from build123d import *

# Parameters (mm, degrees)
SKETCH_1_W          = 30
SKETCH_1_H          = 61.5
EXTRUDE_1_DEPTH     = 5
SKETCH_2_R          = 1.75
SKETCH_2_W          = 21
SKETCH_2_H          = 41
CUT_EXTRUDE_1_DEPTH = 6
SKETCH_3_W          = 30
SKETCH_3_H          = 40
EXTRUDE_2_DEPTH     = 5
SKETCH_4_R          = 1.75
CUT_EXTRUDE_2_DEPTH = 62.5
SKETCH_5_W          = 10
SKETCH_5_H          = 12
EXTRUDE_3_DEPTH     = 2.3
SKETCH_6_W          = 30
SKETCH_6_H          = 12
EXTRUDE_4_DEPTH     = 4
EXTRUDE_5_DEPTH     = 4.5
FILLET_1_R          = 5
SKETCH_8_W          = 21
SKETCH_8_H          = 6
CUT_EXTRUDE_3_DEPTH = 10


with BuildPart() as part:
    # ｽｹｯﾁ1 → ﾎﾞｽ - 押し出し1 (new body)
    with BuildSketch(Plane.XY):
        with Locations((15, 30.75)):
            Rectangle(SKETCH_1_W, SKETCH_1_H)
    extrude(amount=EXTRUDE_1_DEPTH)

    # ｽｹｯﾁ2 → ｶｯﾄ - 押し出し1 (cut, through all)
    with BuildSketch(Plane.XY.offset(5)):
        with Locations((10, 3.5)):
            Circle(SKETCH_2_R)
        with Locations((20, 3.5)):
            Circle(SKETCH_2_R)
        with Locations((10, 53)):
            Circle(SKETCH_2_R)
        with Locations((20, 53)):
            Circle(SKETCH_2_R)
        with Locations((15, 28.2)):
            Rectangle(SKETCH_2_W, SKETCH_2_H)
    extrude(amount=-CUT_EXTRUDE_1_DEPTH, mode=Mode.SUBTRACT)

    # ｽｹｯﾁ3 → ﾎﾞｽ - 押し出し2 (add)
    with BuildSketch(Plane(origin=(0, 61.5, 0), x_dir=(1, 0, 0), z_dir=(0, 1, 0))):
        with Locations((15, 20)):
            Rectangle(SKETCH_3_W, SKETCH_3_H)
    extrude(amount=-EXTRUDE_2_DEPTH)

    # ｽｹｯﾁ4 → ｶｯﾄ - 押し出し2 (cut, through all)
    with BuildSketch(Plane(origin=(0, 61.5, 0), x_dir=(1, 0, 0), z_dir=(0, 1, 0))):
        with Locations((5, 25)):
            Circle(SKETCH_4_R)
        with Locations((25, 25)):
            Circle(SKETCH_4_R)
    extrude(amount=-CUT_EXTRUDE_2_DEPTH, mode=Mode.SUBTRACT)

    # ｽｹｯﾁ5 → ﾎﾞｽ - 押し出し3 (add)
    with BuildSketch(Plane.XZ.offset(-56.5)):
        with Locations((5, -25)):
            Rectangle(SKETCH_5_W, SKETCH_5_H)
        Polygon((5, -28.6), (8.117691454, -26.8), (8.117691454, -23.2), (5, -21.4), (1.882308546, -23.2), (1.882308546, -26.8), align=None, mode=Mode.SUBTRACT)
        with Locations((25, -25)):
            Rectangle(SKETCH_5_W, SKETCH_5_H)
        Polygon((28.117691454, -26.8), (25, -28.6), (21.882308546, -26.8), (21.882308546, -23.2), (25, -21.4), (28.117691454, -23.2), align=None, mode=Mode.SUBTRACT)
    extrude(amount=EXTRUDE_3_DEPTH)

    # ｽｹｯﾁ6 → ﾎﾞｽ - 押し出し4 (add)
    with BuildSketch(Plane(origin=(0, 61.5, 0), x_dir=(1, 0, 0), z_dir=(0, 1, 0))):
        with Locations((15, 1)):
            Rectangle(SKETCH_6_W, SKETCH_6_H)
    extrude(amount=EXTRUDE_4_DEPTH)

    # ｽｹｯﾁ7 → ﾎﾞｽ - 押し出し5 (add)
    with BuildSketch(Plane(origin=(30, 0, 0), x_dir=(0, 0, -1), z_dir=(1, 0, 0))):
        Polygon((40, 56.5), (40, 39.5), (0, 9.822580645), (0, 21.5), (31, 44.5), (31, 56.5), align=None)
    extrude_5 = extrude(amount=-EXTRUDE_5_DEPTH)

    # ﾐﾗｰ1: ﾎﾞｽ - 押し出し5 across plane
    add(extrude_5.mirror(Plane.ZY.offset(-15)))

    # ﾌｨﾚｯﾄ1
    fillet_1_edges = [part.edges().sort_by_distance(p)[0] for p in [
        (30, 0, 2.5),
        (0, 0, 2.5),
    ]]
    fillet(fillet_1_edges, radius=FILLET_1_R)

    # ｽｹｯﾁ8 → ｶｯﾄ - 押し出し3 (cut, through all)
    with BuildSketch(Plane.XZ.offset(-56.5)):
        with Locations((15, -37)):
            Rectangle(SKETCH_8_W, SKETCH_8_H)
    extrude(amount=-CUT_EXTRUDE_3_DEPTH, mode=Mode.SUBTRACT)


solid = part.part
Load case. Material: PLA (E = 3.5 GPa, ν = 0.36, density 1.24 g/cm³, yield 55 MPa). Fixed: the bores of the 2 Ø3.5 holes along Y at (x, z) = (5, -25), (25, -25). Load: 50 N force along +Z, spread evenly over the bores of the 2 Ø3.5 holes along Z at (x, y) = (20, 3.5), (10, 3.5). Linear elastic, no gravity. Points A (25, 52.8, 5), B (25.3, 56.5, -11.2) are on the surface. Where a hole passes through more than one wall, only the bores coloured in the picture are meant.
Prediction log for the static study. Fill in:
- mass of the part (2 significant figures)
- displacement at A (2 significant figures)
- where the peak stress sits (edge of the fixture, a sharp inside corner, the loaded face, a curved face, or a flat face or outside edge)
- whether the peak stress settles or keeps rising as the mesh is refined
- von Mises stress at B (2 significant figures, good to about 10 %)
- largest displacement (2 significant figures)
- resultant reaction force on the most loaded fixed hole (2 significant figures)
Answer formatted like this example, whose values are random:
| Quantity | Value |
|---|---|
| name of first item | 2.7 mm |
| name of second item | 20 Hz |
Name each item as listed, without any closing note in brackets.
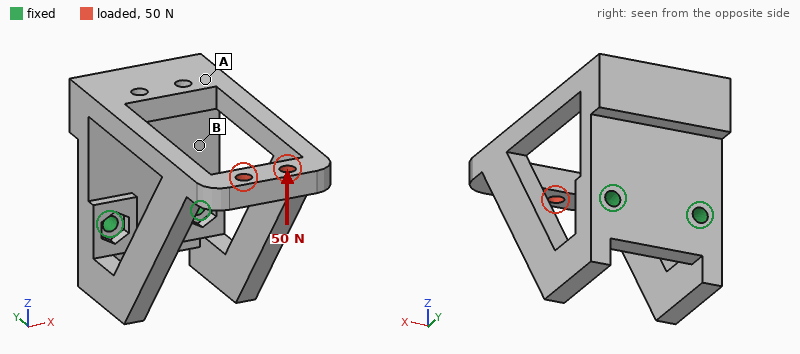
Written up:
| Quantity | Value |
|---|---|
| mass of the part | 21 g |
| displacement at A | 0.36 mm |
| where the peak stress sits | edge of the fixture |
| whether the peak stress settles or keeps rising as the mesh is refined | keeps rising |
| von Mises stress at B | 4.5 MPa |
| largest displacement | 0.88 mm |
| resultant reaction force on the most loaded fixed hole | 25 N |
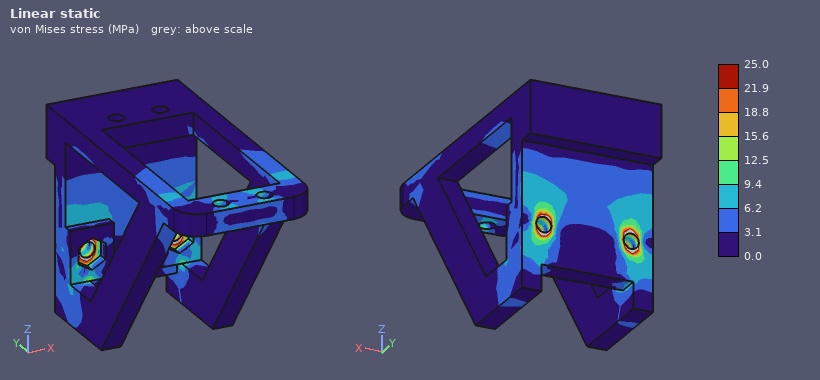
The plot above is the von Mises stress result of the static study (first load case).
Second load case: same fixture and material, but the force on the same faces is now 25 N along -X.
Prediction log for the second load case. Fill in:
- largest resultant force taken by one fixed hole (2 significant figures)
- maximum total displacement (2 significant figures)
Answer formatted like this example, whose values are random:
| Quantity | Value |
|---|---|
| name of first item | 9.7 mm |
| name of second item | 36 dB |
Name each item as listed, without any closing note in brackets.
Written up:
| Quantity | Value |
|---|---|
| largest resultant force taken by one fixed hole | 65 N |
| maximum total displacement | 0.92 mm |
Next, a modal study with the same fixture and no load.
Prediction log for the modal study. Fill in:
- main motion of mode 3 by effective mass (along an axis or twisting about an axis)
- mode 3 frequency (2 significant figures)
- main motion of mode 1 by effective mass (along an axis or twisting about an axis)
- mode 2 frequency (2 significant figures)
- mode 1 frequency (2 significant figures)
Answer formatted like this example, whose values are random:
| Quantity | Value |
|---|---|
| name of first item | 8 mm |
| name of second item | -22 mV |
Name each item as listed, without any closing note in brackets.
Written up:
| Quantity | Value |
|---|---|
| main motion of mode 3 by effective mass | twisting about Y |
| mode 3 frequency | 1300 Hz |
| main motion of mode 1 by effective mass | along X |
| mode 2 frequency | 560 Hz |
| mode 1 frequency | 460 Hz |
